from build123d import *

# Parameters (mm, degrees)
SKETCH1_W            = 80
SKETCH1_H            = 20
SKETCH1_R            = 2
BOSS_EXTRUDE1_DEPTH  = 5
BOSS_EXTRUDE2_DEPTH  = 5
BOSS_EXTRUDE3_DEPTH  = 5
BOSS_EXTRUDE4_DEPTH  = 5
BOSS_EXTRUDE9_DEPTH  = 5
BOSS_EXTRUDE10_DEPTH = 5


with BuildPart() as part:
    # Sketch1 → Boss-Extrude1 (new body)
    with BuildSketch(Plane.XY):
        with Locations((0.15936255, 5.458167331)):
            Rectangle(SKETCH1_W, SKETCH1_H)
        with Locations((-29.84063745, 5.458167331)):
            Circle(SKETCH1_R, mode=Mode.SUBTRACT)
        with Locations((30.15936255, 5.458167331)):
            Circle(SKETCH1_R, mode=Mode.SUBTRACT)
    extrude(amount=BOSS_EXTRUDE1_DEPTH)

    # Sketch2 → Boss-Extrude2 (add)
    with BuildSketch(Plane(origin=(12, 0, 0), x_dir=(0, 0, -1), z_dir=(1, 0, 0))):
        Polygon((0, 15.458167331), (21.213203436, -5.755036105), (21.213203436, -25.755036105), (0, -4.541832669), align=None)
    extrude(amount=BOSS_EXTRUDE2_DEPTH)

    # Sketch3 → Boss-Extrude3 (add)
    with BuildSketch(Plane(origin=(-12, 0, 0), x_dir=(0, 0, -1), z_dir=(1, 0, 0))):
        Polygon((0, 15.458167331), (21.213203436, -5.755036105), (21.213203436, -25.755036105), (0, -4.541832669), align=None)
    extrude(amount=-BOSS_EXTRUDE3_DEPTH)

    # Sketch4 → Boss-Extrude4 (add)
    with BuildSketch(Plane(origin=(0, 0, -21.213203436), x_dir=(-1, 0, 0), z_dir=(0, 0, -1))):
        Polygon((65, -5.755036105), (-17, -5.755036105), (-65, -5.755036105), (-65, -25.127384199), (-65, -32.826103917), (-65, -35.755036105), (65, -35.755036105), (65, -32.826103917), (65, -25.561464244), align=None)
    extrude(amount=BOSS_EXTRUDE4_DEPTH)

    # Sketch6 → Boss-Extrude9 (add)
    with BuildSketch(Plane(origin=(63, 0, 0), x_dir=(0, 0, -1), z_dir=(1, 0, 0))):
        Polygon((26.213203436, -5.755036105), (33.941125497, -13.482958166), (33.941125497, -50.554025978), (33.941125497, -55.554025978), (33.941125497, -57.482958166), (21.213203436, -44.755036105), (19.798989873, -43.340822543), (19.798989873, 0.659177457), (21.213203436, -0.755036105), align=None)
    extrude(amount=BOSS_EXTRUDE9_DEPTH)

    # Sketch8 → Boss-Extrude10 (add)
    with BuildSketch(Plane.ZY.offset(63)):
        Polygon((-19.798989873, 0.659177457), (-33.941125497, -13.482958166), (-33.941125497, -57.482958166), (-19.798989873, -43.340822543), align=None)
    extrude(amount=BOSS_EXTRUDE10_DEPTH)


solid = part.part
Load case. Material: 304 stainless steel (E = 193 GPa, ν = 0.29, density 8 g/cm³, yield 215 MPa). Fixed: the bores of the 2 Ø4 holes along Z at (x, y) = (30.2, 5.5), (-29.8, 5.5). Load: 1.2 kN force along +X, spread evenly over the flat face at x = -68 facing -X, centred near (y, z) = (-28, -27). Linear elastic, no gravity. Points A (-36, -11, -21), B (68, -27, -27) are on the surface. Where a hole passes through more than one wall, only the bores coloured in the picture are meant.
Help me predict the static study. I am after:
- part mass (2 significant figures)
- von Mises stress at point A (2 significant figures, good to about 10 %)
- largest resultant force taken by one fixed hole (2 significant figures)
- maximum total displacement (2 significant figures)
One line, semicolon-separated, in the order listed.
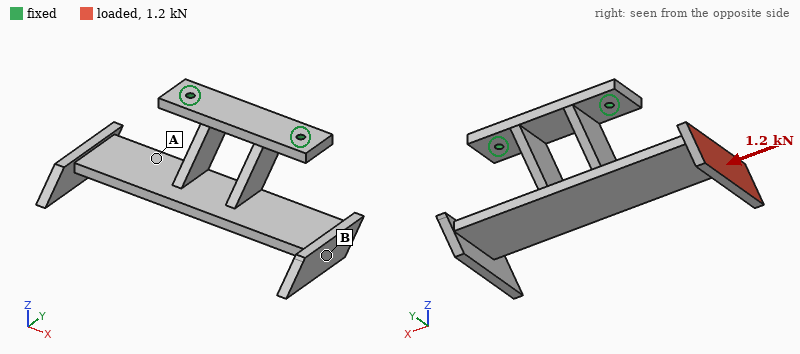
300 g; 28 MPa; 1.2 kN; 0.22 mm
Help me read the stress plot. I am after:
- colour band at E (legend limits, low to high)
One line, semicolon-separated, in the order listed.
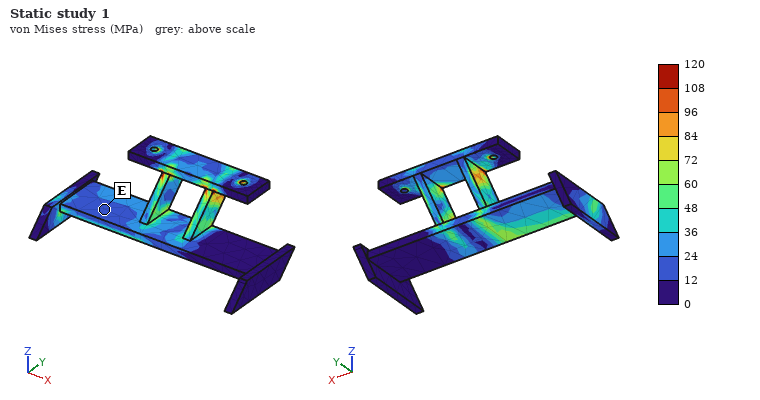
12 to 24 MPa
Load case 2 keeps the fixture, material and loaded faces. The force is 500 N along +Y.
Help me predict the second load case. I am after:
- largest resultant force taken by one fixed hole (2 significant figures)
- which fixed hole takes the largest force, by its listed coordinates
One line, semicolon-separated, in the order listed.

870 N; (-29.8, 5.5)
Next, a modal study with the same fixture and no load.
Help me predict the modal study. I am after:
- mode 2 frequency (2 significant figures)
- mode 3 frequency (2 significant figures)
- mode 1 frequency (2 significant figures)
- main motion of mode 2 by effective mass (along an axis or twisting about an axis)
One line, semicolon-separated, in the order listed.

600 Hz; 1000 Hz; 570 Hz; along Z
